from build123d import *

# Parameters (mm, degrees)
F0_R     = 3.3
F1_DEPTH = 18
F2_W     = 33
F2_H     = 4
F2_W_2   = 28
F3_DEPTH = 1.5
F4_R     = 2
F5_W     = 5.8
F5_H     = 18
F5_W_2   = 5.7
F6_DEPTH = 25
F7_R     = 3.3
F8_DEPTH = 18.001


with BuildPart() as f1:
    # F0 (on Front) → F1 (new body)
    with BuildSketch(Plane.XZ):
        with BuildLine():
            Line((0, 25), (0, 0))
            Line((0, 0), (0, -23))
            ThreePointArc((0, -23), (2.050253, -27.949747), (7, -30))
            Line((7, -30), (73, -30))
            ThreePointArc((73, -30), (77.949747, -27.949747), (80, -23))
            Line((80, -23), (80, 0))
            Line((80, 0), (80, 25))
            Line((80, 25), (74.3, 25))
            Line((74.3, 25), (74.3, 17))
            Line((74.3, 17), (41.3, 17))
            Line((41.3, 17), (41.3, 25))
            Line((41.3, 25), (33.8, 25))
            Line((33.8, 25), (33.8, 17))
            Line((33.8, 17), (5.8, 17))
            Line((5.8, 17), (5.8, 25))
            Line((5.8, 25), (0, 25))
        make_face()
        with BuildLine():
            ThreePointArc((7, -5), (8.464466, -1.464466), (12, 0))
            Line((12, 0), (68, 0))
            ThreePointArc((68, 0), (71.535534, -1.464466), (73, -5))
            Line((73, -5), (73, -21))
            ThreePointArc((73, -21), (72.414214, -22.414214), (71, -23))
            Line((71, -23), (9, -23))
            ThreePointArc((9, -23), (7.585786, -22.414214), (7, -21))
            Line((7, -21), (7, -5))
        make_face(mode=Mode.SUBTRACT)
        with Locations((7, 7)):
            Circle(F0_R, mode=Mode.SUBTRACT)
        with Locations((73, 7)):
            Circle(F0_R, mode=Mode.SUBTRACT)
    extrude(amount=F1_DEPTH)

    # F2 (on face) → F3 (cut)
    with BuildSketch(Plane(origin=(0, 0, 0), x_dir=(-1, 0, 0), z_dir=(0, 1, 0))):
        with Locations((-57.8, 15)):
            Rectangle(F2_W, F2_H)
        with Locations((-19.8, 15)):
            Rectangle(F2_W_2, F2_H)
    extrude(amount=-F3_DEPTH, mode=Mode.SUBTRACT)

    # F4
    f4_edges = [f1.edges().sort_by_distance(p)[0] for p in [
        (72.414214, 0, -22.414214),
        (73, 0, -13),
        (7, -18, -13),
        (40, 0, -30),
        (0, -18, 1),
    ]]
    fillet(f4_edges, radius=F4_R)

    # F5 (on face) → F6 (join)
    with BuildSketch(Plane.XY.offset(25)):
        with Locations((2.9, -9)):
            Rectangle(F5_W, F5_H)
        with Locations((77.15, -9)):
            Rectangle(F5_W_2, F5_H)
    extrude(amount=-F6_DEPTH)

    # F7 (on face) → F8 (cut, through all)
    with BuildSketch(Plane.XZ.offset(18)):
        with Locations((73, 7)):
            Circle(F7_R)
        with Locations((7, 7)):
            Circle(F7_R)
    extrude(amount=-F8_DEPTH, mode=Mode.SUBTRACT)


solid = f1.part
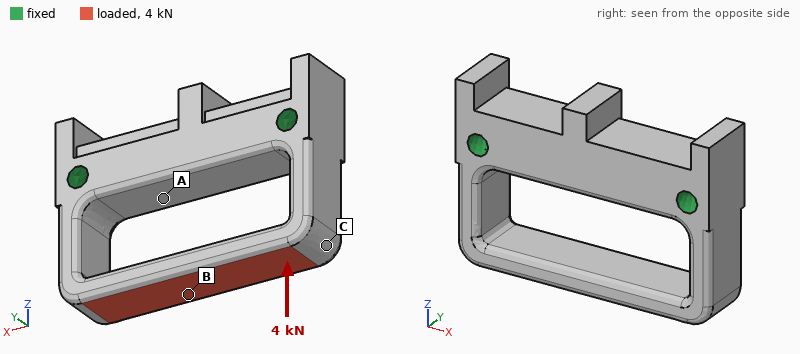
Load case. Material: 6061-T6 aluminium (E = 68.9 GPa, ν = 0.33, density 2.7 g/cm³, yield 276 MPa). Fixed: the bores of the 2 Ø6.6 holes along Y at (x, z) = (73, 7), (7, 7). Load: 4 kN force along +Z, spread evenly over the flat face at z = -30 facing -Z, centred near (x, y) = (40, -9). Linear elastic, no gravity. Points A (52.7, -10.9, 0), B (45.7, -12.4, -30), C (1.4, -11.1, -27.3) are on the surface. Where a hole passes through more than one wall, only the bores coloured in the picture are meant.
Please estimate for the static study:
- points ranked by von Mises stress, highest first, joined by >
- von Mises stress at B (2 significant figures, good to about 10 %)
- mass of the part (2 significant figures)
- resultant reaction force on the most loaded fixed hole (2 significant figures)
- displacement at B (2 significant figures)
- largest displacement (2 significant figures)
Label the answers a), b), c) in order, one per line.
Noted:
a) B > C > A
b) 120 MPa
c) 110 g
d) 2.3 kN
e) 0.20 mm
f) 0.21 mm
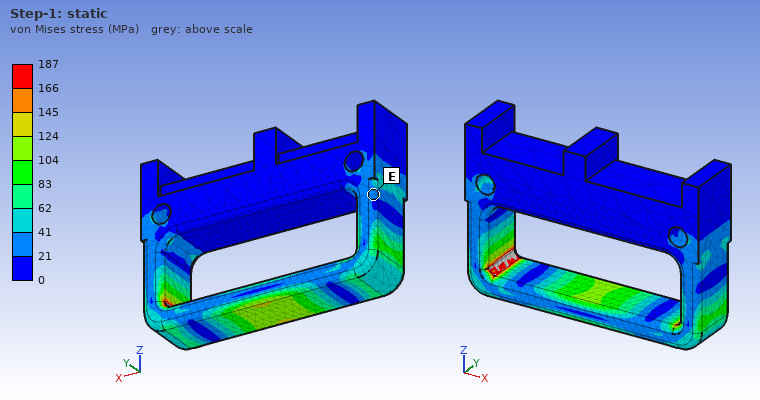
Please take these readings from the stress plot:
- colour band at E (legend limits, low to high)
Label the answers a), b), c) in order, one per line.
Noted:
a) 21 to 41 MPa
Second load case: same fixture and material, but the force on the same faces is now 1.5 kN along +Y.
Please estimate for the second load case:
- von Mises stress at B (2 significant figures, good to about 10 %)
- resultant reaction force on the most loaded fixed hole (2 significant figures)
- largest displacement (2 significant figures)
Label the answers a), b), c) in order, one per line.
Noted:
a) 13 MPa
b) 750 N
c) 96 µm
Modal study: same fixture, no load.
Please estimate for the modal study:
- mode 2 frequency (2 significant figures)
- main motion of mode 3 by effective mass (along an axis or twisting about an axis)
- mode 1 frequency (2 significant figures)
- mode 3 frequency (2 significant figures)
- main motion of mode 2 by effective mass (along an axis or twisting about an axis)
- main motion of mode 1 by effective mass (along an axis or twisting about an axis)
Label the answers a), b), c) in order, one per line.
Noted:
a) 4700 Hz
b) along Z
c) 4100 Hz
d) 5300 Hz
e) along Y
f) along X
